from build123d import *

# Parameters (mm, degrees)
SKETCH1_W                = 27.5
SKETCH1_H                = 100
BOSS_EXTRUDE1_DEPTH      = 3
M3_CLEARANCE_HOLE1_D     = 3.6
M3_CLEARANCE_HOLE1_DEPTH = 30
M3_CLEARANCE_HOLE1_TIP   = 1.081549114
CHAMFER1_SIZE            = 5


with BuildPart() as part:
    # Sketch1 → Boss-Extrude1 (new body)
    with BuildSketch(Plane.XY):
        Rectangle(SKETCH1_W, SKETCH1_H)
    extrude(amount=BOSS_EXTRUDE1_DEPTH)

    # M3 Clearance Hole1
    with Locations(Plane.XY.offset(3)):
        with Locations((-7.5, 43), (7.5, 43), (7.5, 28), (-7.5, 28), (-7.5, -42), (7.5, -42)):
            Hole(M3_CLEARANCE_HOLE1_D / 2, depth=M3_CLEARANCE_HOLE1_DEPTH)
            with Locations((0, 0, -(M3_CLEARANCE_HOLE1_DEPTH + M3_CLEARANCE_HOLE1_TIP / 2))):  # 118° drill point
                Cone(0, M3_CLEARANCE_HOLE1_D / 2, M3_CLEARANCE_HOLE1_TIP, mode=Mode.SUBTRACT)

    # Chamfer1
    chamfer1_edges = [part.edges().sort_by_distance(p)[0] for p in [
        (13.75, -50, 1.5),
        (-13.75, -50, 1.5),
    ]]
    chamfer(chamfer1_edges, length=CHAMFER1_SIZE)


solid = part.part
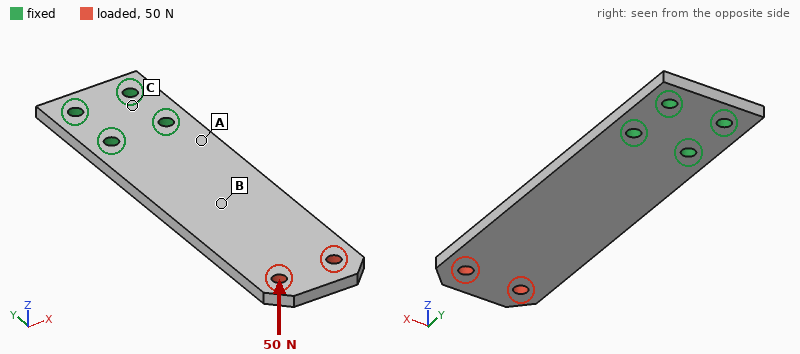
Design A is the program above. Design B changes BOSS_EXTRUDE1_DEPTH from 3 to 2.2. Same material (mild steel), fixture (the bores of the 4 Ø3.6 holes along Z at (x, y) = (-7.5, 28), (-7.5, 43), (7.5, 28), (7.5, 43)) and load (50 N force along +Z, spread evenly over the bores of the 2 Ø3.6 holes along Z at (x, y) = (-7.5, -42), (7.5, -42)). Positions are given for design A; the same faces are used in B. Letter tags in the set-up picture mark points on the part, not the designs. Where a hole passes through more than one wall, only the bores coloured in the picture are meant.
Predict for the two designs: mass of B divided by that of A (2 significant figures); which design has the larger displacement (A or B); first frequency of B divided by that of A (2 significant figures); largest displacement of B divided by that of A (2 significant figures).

0.73
B
0.74
2.5
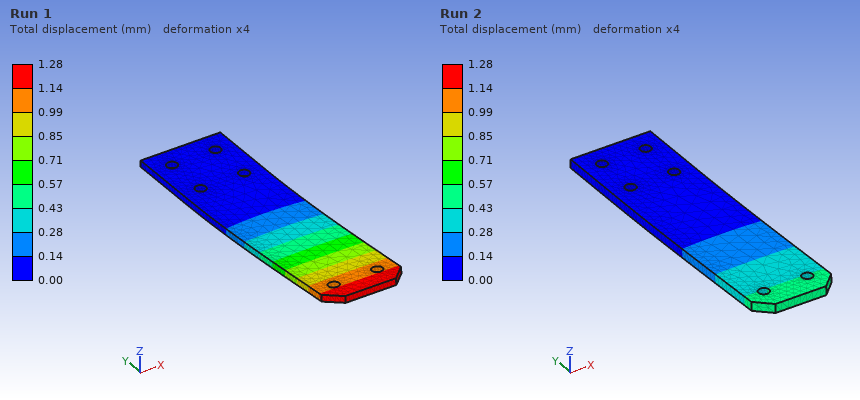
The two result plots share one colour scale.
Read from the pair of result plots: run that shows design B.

Run 1
